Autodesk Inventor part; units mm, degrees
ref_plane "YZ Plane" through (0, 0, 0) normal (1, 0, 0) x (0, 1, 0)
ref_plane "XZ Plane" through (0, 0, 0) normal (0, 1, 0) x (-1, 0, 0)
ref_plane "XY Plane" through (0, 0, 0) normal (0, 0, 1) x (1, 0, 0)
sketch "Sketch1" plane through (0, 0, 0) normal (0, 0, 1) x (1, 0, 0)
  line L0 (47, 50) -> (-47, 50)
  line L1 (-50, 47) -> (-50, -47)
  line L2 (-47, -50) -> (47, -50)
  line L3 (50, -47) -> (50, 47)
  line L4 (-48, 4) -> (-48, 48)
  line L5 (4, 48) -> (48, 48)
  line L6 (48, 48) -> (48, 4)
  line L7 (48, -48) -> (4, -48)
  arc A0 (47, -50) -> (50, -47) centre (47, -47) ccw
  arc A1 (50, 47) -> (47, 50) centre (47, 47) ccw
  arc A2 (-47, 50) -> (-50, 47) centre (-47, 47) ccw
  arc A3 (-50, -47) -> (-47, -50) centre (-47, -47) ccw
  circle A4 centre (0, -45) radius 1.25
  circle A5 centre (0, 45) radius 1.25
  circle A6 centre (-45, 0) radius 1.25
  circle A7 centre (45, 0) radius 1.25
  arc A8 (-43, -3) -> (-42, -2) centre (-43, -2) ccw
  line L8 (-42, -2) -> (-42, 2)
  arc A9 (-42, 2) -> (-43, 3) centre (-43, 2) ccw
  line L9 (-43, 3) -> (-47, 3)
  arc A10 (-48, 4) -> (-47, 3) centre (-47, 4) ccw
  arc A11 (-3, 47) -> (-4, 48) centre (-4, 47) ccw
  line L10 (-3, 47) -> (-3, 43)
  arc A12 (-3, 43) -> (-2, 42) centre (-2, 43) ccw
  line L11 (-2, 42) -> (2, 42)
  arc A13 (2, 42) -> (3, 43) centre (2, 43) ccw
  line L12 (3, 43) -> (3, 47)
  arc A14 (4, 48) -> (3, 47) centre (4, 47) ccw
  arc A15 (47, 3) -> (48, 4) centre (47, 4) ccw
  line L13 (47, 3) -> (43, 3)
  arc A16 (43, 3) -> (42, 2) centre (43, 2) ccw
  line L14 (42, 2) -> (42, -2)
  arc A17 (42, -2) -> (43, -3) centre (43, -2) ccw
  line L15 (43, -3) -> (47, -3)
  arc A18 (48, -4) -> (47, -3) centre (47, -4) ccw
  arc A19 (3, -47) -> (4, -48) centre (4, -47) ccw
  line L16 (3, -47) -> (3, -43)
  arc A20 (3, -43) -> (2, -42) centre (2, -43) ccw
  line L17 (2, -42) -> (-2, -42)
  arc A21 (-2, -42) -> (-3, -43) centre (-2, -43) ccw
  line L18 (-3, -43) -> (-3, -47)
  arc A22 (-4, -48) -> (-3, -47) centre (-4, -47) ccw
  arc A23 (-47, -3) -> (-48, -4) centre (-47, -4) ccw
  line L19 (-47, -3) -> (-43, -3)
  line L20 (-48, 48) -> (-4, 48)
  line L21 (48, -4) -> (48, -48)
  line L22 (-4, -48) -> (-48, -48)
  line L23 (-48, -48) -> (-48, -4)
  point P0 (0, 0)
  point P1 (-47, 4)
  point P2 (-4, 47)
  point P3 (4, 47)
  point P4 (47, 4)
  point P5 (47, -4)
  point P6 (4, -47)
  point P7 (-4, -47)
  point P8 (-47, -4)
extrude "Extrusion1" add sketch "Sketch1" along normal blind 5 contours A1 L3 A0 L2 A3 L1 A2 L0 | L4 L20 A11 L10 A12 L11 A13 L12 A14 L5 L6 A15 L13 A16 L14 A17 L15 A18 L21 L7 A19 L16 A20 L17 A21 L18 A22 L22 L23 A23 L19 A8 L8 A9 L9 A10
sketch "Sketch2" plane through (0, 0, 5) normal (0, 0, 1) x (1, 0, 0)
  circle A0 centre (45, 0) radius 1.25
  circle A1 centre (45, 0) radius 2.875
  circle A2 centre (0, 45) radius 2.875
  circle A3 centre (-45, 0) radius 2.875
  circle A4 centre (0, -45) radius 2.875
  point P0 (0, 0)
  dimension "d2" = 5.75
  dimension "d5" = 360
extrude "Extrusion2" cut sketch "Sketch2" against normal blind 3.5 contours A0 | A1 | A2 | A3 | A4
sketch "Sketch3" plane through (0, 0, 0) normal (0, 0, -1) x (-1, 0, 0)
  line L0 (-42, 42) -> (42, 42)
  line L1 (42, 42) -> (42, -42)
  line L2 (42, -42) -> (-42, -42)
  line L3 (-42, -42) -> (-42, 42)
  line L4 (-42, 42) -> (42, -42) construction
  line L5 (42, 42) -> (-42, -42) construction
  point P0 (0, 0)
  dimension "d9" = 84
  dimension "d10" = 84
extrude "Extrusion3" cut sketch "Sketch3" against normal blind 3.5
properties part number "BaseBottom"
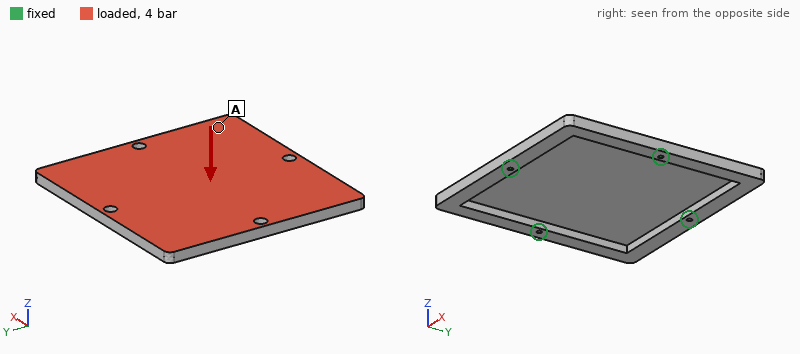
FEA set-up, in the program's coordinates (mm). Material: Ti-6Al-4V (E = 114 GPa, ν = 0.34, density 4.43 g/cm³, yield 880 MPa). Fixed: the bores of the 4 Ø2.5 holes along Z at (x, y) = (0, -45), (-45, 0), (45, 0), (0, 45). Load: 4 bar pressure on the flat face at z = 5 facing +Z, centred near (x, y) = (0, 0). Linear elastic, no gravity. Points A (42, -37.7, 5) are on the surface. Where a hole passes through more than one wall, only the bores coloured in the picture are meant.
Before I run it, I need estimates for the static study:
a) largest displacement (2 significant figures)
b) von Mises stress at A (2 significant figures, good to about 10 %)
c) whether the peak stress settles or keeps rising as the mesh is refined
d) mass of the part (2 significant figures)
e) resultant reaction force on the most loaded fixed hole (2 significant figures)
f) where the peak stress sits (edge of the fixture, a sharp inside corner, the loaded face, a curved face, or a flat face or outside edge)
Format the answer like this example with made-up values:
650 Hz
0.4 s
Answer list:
0.81 mm
45 MPa
keeps rising
110 g
1.5 kN
edge of the fixture
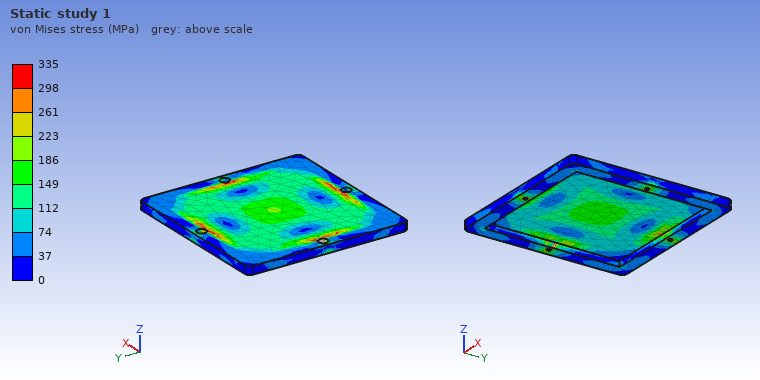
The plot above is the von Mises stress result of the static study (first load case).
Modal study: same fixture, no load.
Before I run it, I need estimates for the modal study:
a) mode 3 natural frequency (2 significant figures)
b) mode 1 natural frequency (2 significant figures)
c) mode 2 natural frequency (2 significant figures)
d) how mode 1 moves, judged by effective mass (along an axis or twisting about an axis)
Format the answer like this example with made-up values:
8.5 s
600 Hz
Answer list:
1900 Hz
1700 Hz
1900 Hz
along Z
